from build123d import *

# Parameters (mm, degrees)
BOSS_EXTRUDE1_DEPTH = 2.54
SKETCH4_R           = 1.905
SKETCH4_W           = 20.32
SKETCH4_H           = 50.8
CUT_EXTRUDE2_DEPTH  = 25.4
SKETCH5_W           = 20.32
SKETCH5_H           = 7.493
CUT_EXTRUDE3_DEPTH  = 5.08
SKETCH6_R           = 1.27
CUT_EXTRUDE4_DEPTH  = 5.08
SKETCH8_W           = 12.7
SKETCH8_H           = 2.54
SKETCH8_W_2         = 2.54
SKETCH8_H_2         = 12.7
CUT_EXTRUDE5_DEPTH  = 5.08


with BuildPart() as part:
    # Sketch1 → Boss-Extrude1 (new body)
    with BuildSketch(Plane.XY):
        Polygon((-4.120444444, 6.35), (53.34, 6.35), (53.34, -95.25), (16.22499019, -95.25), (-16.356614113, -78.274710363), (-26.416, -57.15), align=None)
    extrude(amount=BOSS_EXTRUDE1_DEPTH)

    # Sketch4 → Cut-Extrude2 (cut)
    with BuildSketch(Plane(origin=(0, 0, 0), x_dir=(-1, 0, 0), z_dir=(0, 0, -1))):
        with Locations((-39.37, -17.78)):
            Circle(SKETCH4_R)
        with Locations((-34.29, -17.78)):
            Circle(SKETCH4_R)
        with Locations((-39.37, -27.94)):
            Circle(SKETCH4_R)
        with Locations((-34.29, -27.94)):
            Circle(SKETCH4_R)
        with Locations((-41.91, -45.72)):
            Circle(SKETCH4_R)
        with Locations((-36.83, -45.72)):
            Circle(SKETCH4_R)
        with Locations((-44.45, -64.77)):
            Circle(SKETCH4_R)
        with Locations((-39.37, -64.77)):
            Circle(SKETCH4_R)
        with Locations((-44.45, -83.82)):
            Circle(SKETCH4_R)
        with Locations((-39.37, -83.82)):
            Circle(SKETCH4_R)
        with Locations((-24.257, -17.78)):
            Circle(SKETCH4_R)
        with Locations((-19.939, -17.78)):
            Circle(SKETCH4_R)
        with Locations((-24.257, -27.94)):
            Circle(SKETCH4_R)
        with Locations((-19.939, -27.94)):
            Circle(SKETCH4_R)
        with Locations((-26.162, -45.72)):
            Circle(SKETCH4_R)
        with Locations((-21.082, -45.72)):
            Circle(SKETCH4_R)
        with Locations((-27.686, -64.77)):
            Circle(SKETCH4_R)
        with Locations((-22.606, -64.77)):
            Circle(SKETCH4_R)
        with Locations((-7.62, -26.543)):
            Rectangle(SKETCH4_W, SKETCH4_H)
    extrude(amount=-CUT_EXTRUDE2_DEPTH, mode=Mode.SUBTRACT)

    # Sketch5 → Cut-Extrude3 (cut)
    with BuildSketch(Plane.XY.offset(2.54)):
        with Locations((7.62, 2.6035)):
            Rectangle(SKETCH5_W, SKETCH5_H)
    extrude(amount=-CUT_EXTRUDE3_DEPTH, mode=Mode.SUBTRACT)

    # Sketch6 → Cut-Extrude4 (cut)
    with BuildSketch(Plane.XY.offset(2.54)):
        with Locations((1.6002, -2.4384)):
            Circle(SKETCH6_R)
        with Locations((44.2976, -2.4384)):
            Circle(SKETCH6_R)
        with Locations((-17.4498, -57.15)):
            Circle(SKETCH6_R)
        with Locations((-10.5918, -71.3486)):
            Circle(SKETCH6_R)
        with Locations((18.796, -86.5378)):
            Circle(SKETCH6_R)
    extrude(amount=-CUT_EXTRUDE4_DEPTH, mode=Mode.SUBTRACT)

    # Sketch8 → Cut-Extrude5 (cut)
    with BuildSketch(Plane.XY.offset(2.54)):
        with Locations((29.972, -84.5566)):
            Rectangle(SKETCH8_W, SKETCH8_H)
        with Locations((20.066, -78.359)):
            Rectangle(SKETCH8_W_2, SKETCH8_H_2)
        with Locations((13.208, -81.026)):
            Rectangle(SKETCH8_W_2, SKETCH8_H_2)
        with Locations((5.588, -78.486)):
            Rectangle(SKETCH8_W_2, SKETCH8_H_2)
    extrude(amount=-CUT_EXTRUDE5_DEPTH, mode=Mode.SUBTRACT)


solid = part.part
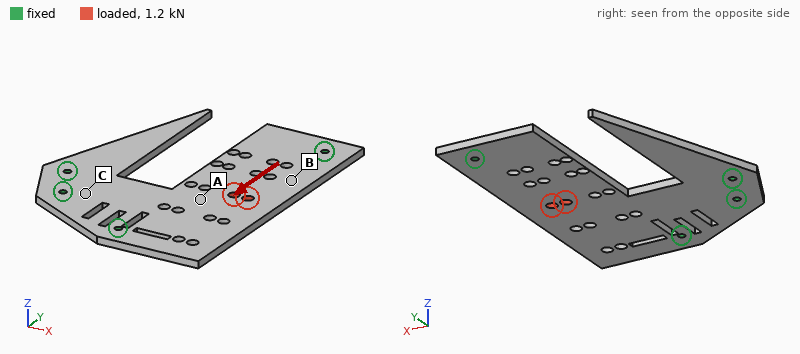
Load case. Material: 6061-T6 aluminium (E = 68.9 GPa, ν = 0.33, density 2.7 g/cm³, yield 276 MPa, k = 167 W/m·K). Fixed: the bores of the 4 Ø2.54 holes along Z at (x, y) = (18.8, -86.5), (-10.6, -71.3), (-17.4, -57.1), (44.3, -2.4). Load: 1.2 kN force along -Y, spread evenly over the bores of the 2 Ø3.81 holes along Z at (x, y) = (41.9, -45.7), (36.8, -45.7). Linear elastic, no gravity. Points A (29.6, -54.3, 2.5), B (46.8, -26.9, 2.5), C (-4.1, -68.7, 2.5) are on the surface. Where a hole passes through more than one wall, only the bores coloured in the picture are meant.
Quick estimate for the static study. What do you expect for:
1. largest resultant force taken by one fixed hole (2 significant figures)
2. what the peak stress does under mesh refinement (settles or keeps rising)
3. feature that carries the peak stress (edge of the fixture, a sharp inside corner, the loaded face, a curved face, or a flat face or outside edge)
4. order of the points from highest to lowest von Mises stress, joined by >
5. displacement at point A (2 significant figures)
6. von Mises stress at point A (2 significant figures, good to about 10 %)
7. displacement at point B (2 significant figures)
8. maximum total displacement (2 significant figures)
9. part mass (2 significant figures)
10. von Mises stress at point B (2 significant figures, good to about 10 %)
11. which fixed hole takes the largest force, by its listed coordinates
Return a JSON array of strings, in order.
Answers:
["760 N", "keeps rising", "edge of the fixture", "B > A > C", "9.8 µm", "7.3 MPa", "8.3 µm", "15 µm", "36 g", "18 MPa", "(44.3, -2.4)"]
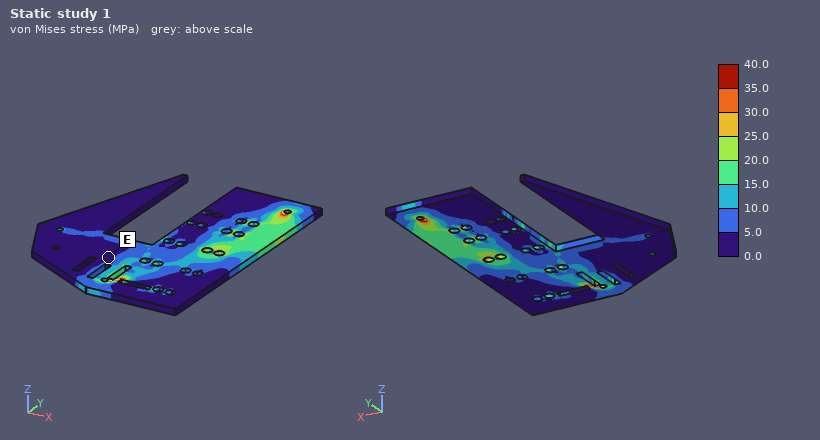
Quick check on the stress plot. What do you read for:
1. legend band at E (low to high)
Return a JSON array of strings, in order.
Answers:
["0.0 to 5.0 MPa"]
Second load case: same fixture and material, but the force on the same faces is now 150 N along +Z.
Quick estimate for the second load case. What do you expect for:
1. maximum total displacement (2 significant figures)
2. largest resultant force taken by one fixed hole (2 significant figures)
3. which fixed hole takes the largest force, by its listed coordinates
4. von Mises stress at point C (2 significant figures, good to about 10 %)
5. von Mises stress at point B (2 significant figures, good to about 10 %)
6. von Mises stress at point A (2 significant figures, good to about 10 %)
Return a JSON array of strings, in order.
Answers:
["0.35 mm", "75 N", "(44.3, -2.4)", "16 MPa", "19 MPa", "22 MPa"]
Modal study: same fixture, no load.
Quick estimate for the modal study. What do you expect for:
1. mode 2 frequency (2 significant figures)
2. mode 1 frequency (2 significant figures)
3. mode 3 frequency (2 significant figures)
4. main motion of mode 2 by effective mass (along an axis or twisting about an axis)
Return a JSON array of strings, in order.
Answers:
["1200 Hz", "890 Hz", "2000 Hz", "along Z"]
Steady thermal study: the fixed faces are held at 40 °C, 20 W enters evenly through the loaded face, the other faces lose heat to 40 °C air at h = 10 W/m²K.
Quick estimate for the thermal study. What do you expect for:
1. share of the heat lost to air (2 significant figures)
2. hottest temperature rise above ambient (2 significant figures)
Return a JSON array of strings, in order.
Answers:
["8.0 %", "45 K"]
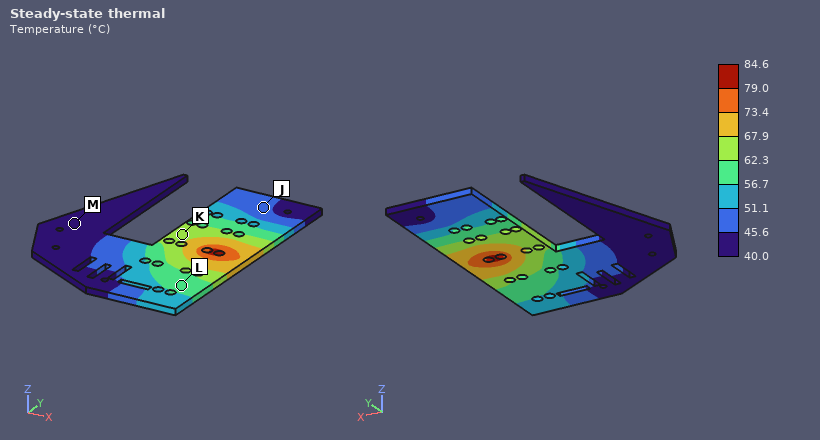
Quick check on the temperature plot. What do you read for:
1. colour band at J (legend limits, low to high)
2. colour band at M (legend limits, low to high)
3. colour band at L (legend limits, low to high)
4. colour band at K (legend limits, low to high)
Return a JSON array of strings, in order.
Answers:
["45.6 to 51.1 °C", "40.0 to 45.6 °C", "56.7 to 62.3 °C", "62.3 to 67.9 °C"]
